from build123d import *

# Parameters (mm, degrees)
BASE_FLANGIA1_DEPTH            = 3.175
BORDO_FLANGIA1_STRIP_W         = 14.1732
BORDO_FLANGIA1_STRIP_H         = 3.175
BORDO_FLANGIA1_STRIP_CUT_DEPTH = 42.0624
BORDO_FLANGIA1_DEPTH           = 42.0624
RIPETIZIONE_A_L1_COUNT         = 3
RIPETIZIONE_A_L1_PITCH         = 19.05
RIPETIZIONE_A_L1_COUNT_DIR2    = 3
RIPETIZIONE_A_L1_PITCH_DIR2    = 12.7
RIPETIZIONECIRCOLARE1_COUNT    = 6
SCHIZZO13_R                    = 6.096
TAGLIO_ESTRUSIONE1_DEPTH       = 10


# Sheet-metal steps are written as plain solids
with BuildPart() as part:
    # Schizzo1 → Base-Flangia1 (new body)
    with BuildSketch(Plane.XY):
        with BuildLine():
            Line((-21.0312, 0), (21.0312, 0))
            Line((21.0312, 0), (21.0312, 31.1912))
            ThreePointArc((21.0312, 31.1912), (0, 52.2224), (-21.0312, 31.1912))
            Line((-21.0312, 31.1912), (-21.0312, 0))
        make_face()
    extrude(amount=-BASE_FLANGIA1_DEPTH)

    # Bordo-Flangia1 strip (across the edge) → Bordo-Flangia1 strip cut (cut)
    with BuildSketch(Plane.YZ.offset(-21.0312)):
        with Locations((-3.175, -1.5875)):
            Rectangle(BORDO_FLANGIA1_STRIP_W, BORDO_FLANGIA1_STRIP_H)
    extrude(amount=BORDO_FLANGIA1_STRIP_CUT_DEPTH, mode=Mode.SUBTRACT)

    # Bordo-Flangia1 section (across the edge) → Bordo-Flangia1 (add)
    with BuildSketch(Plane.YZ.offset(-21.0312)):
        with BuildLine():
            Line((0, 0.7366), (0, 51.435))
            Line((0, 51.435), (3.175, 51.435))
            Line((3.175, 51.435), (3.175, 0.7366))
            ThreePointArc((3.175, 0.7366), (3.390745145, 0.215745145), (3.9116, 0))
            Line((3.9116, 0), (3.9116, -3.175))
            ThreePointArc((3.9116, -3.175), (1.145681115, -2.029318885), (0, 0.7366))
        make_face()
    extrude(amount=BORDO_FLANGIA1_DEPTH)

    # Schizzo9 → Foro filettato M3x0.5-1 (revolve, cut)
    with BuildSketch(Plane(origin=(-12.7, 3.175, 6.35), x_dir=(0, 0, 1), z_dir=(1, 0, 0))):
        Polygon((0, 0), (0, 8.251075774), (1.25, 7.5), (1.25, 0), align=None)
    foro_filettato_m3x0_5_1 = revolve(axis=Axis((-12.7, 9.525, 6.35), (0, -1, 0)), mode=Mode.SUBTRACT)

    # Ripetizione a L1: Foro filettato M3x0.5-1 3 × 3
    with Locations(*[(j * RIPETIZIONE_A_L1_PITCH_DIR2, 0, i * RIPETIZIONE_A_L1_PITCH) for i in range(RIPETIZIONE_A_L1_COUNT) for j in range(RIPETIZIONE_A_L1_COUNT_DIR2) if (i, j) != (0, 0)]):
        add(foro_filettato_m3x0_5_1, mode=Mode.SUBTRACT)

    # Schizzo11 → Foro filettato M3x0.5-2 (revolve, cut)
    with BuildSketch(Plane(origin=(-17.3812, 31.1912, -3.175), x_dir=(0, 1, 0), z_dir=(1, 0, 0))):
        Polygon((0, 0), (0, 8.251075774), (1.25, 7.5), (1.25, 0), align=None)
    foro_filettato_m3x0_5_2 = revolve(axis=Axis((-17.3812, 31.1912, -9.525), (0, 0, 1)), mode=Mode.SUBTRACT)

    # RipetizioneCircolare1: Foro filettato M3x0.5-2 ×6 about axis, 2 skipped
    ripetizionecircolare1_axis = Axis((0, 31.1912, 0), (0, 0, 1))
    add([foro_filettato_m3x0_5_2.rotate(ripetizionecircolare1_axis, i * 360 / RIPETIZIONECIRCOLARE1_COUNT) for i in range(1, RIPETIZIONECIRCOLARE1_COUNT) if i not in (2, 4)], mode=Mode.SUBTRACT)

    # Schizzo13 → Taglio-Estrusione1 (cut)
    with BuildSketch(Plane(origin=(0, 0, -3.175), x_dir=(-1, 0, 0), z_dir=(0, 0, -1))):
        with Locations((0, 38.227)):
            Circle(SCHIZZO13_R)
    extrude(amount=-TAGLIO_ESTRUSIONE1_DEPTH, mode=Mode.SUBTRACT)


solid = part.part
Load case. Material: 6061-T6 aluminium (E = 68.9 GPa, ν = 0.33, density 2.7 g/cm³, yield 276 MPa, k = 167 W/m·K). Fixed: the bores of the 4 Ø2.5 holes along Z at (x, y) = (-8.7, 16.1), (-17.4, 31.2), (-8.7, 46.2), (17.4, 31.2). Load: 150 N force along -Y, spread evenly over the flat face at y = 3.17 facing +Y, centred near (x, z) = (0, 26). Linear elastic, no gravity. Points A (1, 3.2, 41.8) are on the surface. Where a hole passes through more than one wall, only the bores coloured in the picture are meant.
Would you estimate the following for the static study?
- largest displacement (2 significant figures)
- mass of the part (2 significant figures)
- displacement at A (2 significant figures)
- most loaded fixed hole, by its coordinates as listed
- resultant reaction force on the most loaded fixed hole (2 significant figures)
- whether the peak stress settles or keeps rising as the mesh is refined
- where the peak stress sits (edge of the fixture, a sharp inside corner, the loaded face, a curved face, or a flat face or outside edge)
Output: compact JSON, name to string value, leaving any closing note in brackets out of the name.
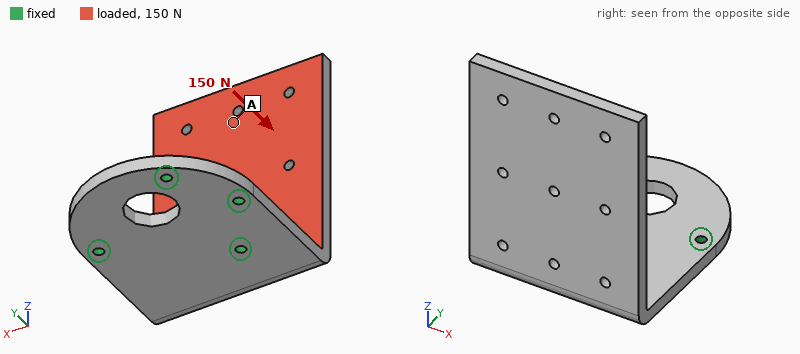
{"largest displacement": "0.84 mm", "mass of the part": "34 g", "displacement at A": "0.66 mm", "most loaded fixed hole, by its coordinates as listed": "(-8.7, 16.1)", "resultant reaction force on the most loaded fixed hole": "170 N", "whether the peak stress settles or keeps rising as the mesh is refined": "keeps rising", "where the peak stress sits": "edge of the fixture"}
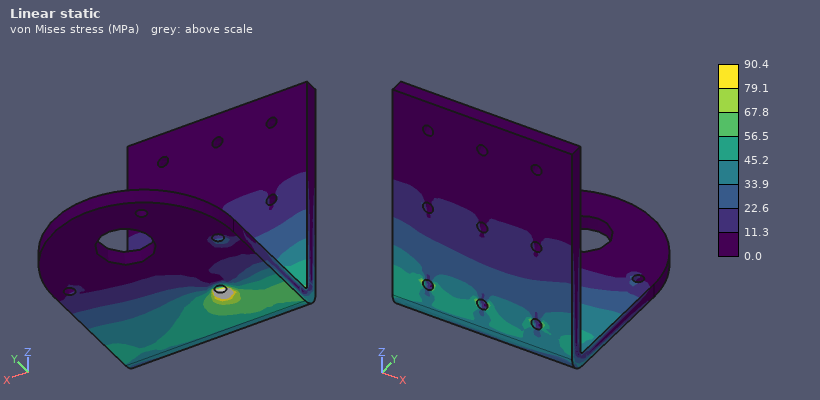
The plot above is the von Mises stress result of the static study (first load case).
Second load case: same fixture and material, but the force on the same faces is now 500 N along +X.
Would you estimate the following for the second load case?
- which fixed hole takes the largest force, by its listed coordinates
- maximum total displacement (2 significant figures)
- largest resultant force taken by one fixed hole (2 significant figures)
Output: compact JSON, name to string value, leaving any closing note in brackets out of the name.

{"which fixed hole takes the largest force, by its listed coordinates": "(-8.7, 16.1)", "maximum total displacement": "1.0 mm", "largest resultant force taken by one fixed hole": "490 N"}
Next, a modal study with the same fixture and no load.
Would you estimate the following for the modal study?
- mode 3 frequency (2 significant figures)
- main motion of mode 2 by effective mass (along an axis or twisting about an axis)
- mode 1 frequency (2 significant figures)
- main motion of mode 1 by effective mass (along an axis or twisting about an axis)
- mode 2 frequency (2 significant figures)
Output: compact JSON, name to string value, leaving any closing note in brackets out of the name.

{"mode 3 frequency": "2400 Hz", "main motion of mode 2 by effective mass": "along X", "mode 1 frequency": "610 Hz", "main motion of mode 1 by effective mass": "along Y", "mode 2 frequency": "1100 Hz"}
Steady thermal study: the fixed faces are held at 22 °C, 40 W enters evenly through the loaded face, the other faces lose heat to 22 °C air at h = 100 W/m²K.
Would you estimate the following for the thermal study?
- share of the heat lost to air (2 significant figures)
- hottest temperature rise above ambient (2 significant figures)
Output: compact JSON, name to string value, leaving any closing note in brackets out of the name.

{"share of the heat lost to air": "40 %", "hottest temperature rise above ambient": "56 K"}
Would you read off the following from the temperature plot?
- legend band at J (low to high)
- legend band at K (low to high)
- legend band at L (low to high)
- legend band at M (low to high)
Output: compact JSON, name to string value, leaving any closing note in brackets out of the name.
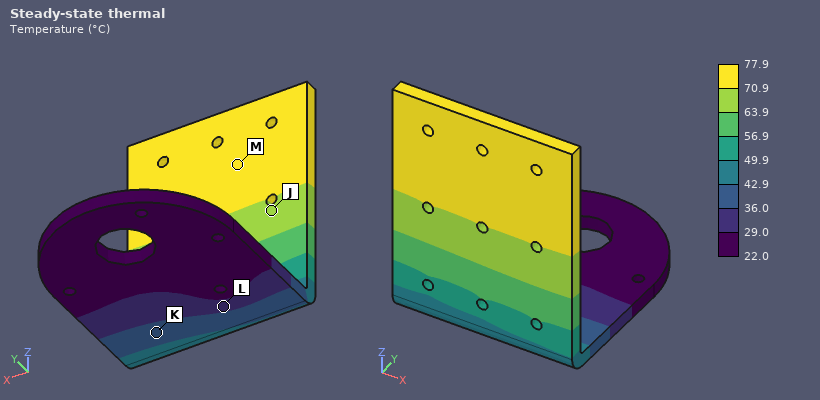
{"legend band at J": "63.9 to 70.9 °C", "legend band at K": "36.0 to 42.9 °C", "legend band at L": "29.0 to 36.0 °C", "legend band at M": "70.9 to 77.9 °C"}
